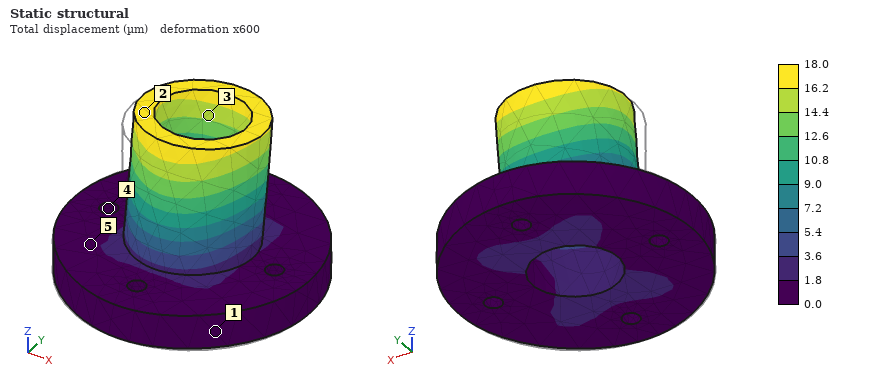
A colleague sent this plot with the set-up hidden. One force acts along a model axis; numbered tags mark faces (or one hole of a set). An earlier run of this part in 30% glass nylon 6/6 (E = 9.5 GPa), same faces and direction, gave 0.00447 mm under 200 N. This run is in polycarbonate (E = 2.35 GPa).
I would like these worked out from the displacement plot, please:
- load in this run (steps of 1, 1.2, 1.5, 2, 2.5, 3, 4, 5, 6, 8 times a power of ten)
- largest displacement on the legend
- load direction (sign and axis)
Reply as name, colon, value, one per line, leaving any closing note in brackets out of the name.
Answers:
load in this run: 200 N
largest displacement on the legend: 18.0 µm
load direction: +Y
